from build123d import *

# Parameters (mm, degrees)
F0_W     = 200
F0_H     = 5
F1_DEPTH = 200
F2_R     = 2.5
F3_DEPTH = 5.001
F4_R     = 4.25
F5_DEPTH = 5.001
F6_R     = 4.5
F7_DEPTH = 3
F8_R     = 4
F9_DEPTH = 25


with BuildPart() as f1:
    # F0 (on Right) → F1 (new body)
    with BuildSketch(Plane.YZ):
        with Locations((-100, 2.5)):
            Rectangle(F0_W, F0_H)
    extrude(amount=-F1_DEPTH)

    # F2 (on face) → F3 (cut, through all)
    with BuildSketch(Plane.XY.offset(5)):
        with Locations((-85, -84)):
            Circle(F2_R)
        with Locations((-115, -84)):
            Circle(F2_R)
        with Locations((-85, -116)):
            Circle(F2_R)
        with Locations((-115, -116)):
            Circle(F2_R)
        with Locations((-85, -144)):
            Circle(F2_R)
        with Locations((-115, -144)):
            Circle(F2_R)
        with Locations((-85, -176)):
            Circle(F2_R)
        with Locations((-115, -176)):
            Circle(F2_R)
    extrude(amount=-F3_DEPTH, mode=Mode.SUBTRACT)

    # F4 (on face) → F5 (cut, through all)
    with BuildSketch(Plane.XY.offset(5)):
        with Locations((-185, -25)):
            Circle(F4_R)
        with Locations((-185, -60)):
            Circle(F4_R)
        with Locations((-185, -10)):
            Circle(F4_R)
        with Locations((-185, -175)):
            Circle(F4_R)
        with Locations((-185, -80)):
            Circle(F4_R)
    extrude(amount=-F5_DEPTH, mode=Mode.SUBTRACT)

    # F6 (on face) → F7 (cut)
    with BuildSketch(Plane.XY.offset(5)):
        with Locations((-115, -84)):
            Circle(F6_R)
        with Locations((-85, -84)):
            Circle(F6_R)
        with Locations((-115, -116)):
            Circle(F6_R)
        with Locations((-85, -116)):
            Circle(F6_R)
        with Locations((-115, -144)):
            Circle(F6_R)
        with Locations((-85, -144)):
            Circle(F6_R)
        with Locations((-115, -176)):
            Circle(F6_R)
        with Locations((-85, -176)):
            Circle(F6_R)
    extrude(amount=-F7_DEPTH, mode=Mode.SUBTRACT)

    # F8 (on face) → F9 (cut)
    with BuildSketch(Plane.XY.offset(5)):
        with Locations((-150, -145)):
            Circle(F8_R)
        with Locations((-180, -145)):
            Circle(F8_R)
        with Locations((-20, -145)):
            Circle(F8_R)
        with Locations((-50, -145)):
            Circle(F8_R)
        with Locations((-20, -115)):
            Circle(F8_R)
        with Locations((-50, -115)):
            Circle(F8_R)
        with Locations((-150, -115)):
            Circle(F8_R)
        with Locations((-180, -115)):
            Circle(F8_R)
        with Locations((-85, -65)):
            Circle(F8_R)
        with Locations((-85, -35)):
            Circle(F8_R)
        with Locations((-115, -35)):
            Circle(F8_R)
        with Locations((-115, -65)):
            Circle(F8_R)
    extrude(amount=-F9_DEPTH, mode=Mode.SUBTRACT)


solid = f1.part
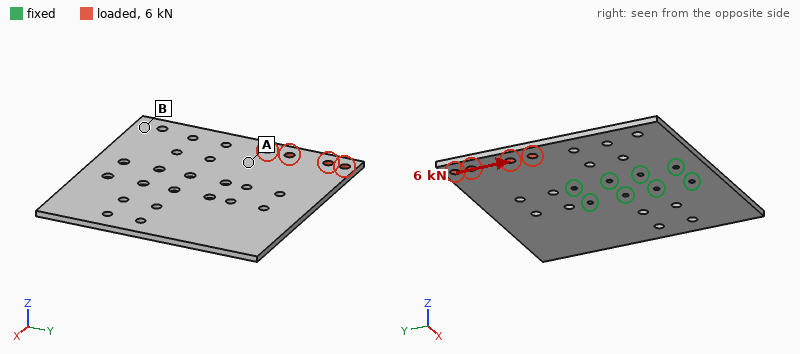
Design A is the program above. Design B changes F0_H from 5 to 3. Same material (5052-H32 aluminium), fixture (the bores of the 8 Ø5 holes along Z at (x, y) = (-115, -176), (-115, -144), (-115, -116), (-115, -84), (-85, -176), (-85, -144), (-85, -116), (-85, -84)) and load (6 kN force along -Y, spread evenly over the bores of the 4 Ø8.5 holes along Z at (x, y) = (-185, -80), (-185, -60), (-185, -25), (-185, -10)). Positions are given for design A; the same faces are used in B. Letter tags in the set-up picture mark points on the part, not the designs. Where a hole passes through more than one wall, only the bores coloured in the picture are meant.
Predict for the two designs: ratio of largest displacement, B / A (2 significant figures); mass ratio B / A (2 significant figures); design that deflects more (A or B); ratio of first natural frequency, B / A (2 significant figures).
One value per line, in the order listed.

1.7
0.60
B
0.61
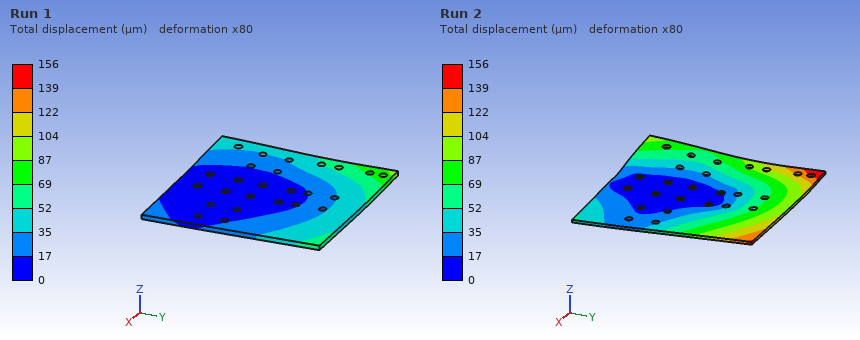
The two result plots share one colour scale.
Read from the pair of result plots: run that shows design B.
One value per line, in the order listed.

Run 2
